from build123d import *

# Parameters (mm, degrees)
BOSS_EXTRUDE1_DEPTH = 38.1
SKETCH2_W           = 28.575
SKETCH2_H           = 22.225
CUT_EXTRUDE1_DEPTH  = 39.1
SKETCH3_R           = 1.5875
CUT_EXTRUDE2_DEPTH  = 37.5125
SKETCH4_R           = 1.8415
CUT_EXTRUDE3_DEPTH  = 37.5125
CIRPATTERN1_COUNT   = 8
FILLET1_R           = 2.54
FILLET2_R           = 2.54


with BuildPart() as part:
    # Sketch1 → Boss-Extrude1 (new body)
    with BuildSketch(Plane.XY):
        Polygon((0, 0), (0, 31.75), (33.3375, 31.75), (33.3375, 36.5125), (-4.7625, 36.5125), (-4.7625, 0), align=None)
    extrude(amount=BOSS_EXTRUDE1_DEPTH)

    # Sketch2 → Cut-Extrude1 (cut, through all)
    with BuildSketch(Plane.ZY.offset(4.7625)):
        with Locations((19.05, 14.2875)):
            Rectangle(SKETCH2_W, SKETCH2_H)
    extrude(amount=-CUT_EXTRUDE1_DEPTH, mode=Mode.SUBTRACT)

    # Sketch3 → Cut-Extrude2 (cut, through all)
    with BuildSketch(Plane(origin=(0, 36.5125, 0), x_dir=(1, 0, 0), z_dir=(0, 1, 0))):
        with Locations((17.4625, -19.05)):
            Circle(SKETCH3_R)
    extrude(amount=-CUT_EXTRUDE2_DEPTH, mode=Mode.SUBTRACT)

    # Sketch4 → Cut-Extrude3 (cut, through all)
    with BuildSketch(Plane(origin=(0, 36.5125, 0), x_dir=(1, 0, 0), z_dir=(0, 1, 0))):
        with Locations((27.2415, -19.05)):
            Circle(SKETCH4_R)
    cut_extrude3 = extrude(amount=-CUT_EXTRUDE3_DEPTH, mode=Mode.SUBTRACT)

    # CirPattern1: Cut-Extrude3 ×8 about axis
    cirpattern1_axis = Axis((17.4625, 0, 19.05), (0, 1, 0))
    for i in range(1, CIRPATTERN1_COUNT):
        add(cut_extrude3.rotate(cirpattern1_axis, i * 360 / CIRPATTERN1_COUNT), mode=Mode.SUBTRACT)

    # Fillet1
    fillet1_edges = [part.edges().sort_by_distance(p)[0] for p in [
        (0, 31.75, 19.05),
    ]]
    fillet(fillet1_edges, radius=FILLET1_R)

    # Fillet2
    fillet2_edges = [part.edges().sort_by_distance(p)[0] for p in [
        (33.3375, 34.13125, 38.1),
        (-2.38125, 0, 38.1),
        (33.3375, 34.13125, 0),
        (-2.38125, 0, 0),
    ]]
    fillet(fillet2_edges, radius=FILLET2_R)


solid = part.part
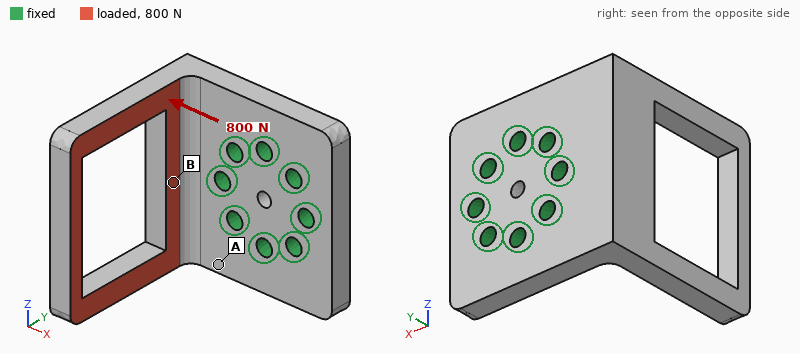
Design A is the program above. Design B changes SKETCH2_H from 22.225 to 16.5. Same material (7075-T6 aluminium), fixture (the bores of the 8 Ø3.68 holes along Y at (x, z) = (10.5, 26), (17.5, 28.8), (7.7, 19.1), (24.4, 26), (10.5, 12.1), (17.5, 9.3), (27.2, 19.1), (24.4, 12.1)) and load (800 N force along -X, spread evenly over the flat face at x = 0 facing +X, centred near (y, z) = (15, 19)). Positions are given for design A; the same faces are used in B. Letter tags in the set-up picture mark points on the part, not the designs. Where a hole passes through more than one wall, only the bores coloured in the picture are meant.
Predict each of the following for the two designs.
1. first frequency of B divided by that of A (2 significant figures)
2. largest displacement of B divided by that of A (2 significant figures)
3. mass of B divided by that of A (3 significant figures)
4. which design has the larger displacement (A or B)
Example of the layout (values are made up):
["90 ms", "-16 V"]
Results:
["0.93", "0.86", "1.08", "A"]
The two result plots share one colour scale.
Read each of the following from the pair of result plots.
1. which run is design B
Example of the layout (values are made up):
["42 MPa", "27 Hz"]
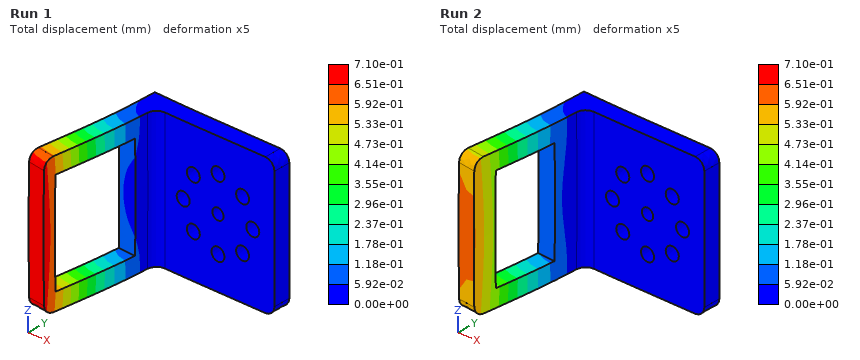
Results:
["Run 2"]
